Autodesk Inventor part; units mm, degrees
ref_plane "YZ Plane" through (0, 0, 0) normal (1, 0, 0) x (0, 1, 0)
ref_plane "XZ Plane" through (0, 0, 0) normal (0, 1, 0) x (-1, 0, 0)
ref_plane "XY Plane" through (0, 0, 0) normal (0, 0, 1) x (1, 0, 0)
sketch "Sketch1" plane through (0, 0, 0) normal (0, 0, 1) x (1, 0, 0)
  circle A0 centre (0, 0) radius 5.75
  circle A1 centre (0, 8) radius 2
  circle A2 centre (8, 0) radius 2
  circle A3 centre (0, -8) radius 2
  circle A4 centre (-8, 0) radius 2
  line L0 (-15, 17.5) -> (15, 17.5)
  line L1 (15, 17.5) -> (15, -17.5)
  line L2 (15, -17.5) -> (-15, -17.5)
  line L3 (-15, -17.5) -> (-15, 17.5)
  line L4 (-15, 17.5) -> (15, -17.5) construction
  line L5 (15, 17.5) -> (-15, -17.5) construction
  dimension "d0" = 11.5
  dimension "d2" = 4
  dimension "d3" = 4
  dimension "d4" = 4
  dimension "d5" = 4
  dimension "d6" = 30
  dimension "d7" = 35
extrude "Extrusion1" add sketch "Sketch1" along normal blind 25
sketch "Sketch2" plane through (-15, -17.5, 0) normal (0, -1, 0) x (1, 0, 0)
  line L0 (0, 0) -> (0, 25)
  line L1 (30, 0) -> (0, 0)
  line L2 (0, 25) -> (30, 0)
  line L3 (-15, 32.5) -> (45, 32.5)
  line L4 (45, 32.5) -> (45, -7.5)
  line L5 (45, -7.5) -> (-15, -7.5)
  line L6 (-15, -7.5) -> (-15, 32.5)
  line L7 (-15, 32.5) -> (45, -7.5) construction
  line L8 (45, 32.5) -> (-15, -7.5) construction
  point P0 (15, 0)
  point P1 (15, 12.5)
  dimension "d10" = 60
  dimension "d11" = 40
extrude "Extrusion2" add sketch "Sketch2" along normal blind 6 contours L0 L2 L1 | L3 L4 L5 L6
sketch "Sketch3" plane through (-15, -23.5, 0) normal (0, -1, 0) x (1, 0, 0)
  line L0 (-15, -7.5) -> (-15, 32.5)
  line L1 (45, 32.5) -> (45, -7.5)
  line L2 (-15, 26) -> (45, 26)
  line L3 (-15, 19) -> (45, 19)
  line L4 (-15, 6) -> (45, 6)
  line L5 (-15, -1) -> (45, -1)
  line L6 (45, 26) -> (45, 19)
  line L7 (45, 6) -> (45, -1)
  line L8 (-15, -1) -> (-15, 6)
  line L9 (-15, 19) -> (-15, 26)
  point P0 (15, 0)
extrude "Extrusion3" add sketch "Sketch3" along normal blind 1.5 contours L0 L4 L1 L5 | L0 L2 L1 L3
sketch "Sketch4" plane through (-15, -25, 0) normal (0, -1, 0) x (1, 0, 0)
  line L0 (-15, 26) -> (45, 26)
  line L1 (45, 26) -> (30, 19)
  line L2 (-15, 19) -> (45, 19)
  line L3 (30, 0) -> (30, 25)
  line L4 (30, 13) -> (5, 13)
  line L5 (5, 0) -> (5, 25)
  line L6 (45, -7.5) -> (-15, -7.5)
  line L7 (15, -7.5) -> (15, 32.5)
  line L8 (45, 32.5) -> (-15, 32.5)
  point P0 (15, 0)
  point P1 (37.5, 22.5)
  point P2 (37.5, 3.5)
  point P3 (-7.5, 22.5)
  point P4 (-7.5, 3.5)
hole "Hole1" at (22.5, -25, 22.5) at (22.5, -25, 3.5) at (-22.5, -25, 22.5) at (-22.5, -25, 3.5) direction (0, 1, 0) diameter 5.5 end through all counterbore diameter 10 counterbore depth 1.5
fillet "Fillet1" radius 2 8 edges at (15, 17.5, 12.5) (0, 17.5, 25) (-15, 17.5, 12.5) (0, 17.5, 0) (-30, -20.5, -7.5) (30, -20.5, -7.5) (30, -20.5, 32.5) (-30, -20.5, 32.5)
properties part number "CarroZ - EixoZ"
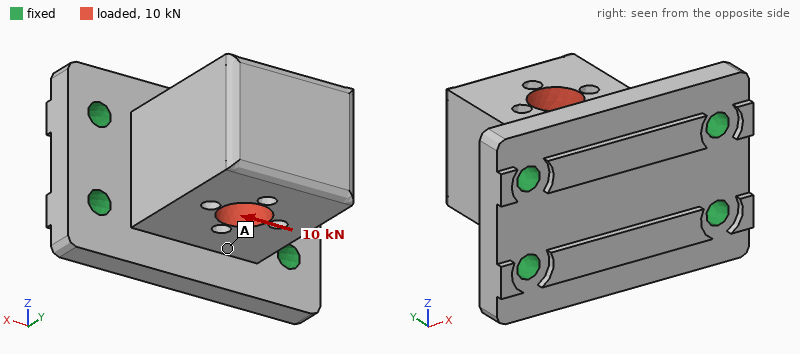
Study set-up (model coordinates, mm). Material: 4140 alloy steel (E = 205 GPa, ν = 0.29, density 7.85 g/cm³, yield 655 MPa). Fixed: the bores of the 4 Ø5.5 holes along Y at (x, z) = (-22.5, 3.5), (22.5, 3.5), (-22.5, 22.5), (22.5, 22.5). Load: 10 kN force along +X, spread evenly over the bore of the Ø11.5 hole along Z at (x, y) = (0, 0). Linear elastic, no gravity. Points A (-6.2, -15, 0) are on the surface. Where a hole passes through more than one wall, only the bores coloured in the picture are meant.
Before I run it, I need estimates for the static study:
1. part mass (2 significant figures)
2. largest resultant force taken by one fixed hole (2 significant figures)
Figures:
290 g
3.9 kN
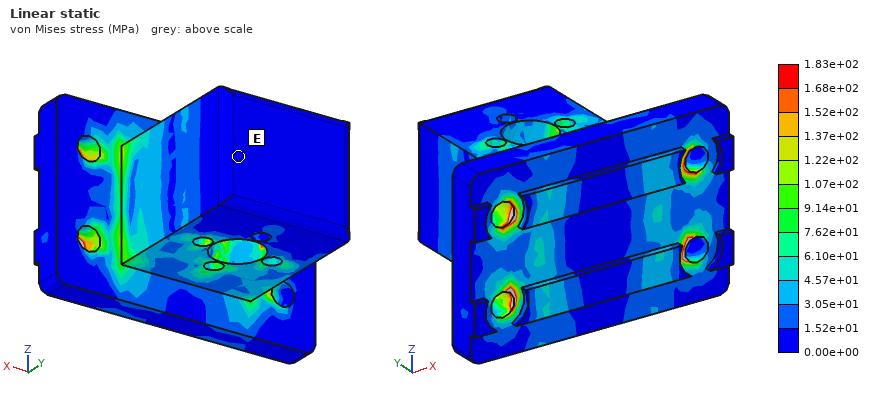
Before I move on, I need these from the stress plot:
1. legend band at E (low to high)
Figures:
0.00e+00 to 1.52e+01 MPa
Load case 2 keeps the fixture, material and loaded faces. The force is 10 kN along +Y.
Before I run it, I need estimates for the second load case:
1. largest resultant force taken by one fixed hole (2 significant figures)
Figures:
2.7 kN
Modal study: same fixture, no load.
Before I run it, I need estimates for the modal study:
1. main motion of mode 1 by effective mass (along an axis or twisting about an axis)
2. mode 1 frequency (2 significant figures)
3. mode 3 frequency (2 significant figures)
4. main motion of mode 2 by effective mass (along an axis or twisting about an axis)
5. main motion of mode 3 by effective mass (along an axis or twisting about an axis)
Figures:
along Z
5400 Hz
12 kHz
along X
along Y
